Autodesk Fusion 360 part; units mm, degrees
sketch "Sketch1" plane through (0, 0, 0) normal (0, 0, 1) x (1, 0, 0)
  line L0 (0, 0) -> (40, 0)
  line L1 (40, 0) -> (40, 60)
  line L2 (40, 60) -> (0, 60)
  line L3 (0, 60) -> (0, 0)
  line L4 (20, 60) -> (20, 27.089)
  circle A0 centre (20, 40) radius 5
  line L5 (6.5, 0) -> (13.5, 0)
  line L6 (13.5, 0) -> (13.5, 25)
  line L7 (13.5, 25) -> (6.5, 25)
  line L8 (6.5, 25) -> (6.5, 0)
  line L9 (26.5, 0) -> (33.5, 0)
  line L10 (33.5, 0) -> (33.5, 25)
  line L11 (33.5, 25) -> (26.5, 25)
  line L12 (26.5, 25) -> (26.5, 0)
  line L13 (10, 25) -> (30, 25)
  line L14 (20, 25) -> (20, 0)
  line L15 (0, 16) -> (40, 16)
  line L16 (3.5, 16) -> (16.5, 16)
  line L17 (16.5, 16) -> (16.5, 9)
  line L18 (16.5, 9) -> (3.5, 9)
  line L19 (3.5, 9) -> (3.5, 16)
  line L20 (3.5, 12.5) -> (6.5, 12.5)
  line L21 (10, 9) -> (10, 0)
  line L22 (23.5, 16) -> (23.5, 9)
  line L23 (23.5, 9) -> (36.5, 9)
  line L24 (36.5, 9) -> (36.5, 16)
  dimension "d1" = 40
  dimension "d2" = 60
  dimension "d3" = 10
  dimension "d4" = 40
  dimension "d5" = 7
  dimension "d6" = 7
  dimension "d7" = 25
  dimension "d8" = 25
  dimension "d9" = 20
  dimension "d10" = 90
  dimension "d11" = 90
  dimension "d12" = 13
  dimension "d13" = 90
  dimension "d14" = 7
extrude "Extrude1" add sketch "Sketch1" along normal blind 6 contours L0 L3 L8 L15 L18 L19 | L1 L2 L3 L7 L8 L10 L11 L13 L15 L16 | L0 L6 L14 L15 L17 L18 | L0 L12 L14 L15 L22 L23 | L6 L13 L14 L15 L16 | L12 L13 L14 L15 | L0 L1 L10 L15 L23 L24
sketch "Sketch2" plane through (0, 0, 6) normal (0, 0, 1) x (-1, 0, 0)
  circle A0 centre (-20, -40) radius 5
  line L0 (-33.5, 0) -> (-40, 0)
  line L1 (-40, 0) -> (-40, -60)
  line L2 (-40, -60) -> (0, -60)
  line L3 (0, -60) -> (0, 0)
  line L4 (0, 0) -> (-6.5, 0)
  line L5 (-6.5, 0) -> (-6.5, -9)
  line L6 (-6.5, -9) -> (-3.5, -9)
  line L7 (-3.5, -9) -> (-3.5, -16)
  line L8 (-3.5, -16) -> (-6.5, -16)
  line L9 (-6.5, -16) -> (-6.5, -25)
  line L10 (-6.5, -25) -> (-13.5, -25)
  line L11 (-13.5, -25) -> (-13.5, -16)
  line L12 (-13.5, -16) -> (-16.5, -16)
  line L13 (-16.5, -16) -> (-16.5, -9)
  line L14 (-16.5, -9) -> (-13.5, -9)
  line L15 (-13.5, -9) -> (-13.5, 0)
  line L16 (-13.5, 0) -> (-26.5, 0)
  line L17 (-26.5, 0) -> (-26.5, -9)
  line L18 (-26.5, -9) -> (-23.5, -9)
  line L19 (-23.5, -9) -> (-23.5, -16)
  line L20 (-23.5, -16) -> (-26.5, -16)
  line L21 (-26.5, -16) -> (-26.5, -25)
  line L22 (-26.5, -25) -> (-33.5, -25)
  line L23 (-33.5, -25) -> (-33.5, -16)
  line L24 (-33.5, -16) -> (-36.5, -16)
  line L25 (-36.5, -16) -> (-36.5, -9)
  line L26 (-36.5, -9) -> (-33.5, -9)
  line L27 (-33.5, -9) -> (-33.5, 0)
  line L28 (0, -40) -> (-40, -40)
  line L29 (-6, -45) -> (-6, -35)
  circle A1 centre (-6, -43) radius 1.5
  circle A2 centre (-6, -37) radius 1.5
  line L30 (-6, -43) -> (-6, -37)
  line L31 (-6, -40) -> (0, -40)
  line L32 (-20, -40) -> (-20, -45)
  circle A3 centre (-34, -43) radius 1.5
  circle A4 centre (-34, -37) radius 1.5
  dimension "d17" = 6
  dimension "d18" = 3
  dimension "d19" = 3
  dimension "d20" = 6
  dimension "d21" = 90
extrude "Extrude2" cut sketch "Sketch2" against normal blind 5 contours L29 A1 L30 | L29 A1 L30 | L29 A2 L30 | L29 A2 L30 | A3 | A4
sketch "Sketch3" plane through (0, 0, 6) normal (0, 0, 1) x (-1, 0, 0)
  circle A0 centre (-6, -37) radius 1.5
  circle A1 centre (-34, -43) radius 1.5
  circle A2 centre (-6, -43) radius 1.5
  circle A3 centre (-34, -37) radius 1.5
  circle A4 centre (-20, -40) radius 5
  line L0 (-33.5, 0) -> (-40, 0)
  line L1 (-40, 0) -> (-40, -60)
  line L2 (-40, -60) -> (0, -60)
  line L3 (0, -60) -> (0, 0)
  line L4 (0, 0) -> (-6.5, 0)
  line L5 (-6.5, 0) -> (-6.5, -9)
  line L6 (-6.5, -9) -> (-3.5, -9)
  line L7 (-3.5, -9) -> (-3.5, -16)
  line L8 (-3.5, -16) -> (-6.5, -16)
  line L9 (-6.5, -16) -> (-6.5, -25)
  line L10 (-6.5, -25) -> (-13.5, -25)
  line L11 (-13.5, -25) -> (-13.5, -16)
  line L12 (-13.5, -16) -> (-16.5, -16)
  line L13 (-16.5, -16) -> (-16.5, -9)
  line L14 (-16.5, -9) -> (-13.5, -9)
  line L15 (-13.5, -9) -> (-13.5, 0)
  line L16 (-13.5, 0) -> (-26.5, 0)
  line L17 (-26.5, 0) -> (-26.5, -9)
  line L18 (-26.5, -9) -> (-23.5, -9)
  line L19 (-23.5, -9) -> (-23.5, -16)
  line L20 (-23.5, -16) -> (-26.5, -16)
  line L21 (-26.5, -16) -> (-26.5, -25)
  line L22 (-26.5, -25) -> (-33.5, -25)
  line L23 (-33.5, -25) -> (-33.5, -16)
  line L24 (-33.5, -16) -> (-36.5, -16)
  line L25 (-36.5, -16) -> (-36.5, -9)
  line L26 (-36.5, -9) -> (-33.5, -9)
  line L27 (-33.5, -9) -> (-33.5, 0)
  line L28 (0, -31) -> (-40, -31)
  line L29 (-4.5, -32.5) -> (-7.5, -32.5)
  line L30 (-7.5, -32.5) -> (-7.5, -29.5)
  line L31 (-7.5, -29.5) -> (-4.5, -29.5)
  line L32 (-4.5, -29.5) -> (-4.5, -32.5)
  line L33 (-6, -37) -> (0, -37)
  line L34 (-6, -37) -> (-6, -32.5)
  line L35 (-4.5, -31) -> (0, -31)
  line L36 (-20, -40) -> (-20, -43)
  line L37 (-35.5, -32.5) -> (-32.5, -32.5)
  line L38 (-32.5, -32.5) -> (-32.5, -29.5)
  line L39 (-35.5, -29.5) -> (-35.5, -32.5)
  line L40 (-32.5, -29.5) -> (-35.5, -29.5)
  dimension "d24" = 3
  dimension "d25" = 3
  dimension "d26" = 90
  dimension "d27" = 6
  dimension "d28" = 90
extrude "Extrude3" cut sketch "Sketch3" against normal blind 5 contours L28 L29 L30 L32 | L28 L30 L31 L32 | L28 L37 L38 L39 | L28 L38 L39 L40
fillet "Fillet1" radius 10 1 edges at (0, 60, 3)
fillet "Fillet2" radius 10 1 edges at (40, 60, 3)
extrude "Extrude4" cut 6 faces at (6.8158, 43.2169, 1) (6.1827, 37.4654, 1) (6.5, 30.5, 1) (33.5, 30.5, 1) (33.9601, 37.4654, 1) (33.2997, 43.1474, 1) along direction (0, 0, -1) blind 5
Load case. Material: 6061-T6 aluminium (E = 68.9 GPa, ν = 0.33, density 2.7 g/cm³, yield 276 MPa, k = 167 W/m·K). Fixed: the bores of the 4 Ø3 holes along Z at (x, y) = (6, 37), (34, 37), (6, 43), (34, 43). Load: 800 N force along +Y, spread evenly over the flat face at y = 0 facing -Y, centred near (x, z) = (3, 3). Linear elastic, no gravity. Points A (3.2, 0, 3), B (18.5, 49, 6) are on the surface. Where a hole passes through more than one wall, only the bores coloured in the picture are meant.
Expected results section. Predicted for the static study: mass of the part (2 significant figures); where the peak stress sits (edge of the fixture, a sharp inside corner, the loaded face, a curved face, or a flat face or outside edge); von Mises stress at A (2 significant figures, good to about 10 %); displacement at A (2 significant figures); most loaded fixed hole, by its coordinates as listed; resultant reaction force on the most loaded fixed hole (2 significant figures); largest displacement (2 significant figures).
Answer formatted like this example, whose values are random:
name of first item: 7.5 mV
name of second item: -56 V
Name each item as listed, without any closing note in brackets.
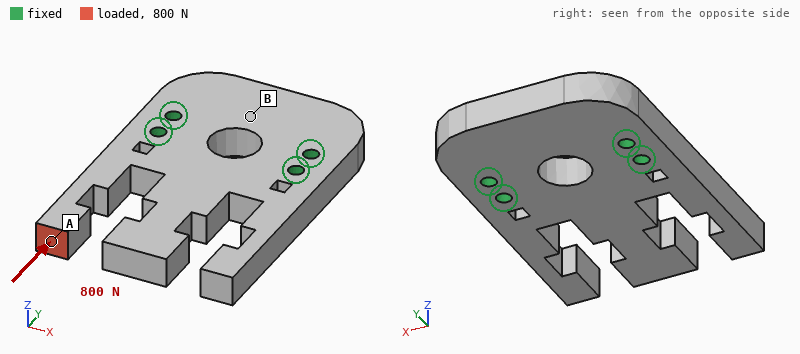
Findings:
mass of the part: 29 g
where the peak stress sits: a flat face or outside edge
von Mises stress at A: 20 MPa
displacement at A: 88 µm
most loaded fixed hole, by its coordinates as listed: (6, 37)
resultant reaction force on the most loaded fixed hole: 620 N
largest displacement: 97 µm
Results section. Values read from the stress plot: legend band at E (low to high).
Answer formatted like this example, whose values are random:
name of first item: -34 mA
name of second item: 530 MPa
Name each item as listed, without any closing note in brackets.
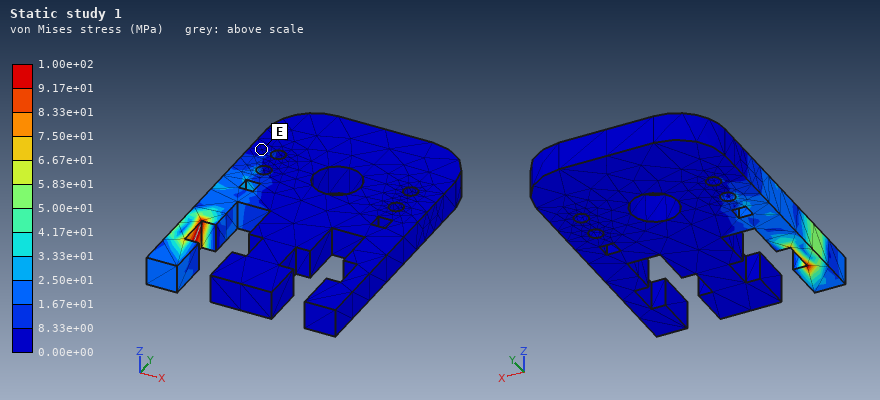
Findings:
legend band at E: 0.00e+00 to 8.33e+00 MPa
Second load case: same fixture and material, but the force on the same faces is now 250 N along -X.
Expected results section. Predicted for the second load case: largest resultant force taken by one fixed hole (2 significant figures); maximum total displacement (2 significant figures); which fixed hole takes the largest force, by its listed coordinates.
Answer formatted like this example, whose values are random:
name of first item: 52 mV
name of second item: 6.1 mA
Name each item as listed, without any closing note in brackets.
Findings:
largest resultant force taken by one fixed hole: 310 N
maximum total displacement: 0.46 mm
which fixed hole takes the largest force, by its listed coordinates: (34, 37)
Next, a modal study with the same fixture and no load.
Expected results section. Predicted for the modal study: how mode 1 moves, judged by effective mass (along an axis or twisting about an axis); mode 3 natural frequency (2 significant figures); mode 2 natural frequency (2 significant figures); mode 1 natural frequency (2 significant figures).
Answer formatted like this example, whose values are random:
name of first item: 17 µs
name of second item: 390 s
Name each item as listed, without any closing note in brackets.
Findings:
how mode 1 moves, judged by effective mass: along Z
mode 3 natural frequency: 4700 Hz
mode 2 natural frequency: 4300 Hz
mode 1 natural frequency: 3600 Hz
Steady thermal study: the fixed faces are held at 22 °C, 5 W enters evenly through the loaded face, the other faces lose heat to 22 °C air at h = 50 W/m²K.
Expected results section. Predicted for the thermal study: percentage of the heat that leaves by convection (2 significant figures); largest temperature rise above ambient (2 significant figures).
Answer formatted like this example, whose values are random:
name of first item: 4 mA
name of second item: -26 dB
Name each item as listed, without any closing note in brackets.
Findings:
percentage of the heat that leaves by convection: 13 %
largest temperature rise above ambient: 29 K
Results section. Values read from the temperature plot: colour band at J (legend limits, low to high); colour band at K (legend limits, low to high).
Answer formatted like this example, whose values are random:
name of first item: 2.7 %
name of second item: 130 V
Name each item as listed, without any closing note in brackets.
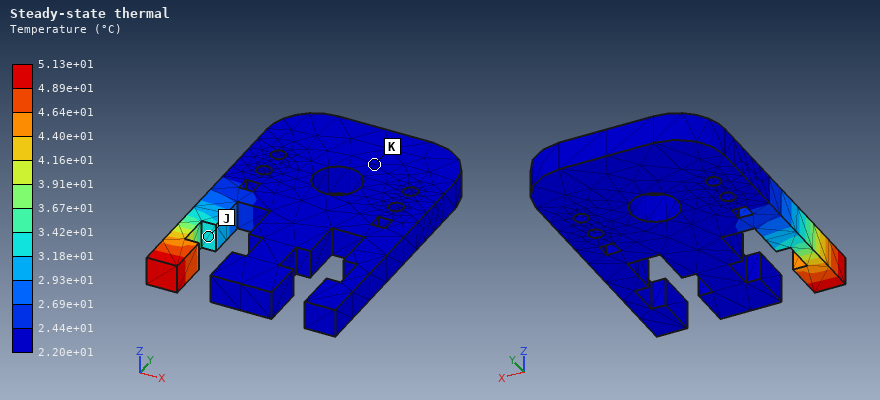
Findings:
colour band at J: 3.18e+01 to 3.42e+01 °C
colour band at K: 2.20e+01 to 2.44e+01 °C
